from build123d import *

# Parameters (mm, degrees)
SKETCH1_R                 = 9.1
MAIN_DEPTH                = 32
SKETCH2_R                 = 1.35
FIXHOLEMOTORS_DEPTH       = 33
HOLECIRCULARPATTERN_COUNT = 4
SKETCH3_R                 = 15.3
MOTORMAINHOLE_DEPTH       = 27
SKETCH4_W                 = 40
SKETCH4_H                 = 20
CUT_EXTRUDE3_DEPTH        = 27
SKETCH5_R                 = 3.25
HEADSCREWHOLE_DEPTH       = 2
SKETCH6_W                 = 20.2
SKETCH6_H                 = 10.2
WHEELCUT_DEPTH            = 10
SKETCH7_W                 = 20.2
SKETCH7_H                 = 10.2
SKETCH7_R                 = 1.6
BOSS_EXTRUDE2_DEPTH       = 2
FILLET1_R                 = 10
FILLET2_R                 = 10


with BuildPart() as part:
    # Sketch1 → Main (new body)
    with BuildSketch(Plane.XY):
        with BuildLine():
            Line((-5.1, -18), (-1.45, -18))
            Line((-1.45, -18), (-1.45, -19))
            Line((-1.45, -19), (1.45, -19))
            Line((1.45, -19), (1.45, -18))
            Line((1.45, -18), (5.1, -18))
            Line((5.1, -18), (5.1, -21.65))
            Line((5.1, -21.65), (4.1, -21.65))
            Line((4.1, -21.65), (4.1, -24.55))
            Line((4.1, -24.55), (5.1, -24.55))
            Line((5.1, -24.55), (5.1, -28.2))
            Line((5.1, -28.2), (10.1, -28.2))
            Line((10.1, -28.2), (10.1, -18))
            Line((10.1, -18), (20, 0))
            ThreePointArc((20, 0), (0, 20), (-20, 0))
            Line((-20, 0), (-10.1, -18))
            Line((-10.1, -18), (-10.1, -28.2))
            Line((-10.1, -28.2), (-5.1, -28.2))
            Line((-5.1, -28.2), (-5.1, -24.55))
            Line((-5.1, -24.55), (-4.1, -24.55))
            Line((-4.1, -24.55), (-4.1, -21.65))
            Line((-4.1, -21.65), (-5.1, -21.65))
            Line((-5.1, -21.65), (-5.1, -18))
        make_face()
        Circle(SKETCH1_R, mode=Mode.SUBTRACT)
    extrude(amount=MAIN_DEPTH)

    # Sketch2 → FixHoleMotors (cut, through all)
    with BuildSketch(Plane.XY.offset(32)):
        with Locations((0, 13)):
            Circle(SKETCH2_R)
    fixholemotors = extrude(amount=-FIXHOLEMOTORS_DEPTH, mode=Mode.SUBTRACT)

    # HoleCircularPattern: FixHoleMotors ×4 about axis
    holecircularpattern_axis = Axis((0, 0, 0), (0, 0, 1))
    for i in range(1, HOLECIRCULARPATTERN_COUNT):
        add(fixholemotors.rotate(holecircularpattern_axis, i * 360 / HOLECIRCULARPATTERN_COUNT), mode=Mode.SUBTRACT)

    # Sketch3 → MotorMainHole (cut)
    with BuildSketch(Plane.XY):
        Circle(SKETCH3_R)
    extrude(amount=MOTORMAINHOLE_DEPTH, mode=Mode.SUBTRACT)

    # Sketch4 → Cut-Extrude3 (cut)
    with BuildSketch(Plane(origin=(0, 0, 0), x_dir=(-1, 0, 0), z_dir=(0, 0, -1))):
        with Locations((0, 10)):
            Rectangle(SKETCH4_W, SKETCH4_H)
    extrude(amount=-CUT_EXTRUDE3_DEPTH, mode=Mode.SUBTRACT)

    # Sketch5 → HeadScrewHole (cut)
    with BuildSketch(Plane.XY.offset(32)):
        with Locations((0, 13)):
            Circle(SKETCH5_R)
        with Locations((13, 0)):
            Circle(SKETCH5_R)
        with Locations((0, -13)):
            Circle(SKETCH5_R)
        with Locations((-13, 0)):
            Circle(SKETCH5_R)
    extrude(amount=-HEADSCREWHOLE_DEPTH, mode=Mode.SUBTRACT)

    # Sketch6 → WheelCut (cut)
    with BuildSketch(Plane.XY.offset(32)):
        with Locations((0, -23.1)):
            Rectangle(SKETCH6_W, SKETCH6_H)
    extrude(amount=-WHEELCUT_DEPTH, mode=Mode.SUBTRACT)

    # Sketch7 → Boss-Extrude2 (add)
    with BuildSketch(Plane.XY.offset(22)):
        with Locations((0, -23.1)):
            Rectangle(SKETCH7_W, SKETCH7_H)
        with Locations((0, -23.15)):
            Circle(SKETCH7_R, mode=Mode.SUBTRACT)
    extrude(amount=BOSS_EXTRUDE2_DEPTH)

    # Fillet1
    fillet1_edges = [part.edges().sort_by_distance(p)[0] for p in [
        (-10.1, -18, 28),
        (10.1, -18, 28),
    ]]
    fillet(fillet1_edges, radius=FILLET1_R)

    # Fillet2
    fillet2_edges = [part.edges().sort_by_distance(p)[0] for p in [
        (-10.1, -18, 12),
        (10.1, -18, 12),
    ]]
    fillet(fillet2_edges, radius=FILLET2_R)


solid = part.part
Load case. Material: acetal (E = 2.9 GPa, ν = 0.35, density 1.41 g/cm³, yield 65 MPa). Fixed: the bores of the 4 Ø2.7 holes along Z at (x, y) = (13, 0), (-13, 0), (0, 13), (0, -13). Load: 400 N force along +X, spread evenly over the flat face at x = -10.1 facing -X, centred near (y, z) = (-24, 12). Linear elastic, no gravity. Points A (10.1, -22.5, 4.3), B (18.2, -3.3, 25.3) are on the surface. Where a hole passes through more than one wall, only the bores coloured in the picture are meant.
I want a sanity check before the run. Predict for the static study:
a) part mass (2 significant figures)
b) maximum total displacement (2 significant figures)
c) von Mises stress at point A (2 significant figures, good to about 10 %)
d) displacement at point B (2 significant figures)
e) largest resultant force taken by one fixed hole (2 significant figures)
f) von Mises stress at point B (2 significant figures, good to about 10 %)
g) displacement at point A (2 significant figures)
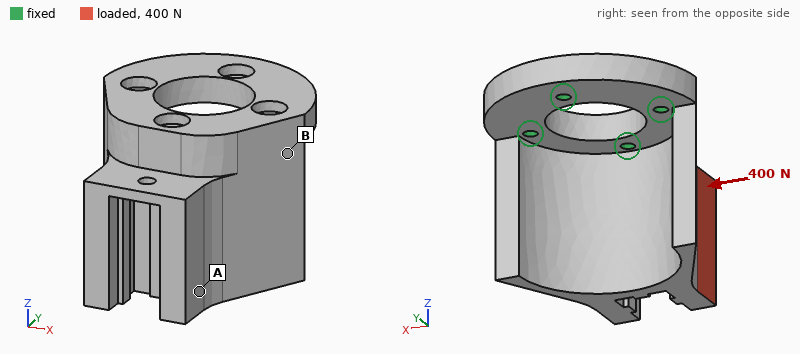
16 g
0.63 mm
3.6 MPa
0.11 mm
310 N
8.3 MPa
0.20 mm
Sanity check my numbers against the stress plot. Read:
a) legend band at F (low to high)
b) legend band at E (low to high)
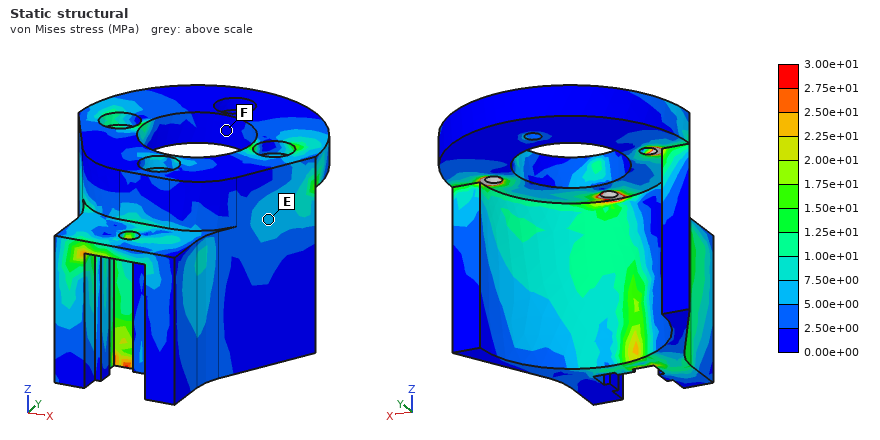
0.00e+00 to 2.50e+00 MPa
5.00e+00 to 7.50e+00 MPa
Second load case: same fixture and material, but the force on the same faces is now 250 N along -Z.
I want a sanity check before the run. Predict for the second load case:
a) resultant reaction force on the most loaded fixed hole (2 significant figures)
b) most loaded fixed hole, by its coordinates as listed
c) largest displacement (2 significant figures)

410 N
(0, -13)
0.62 mm
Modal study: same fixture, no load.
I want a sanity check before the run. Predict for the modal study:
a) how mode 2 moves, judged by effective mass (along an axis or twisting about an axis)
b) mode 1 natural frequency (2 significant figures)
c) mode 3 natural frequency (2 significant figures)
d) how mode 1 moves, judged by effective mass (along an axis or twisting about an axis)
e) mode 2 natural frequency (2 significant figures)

along Y
1300 Hz
2500 Hz
along X
1600 Hz
